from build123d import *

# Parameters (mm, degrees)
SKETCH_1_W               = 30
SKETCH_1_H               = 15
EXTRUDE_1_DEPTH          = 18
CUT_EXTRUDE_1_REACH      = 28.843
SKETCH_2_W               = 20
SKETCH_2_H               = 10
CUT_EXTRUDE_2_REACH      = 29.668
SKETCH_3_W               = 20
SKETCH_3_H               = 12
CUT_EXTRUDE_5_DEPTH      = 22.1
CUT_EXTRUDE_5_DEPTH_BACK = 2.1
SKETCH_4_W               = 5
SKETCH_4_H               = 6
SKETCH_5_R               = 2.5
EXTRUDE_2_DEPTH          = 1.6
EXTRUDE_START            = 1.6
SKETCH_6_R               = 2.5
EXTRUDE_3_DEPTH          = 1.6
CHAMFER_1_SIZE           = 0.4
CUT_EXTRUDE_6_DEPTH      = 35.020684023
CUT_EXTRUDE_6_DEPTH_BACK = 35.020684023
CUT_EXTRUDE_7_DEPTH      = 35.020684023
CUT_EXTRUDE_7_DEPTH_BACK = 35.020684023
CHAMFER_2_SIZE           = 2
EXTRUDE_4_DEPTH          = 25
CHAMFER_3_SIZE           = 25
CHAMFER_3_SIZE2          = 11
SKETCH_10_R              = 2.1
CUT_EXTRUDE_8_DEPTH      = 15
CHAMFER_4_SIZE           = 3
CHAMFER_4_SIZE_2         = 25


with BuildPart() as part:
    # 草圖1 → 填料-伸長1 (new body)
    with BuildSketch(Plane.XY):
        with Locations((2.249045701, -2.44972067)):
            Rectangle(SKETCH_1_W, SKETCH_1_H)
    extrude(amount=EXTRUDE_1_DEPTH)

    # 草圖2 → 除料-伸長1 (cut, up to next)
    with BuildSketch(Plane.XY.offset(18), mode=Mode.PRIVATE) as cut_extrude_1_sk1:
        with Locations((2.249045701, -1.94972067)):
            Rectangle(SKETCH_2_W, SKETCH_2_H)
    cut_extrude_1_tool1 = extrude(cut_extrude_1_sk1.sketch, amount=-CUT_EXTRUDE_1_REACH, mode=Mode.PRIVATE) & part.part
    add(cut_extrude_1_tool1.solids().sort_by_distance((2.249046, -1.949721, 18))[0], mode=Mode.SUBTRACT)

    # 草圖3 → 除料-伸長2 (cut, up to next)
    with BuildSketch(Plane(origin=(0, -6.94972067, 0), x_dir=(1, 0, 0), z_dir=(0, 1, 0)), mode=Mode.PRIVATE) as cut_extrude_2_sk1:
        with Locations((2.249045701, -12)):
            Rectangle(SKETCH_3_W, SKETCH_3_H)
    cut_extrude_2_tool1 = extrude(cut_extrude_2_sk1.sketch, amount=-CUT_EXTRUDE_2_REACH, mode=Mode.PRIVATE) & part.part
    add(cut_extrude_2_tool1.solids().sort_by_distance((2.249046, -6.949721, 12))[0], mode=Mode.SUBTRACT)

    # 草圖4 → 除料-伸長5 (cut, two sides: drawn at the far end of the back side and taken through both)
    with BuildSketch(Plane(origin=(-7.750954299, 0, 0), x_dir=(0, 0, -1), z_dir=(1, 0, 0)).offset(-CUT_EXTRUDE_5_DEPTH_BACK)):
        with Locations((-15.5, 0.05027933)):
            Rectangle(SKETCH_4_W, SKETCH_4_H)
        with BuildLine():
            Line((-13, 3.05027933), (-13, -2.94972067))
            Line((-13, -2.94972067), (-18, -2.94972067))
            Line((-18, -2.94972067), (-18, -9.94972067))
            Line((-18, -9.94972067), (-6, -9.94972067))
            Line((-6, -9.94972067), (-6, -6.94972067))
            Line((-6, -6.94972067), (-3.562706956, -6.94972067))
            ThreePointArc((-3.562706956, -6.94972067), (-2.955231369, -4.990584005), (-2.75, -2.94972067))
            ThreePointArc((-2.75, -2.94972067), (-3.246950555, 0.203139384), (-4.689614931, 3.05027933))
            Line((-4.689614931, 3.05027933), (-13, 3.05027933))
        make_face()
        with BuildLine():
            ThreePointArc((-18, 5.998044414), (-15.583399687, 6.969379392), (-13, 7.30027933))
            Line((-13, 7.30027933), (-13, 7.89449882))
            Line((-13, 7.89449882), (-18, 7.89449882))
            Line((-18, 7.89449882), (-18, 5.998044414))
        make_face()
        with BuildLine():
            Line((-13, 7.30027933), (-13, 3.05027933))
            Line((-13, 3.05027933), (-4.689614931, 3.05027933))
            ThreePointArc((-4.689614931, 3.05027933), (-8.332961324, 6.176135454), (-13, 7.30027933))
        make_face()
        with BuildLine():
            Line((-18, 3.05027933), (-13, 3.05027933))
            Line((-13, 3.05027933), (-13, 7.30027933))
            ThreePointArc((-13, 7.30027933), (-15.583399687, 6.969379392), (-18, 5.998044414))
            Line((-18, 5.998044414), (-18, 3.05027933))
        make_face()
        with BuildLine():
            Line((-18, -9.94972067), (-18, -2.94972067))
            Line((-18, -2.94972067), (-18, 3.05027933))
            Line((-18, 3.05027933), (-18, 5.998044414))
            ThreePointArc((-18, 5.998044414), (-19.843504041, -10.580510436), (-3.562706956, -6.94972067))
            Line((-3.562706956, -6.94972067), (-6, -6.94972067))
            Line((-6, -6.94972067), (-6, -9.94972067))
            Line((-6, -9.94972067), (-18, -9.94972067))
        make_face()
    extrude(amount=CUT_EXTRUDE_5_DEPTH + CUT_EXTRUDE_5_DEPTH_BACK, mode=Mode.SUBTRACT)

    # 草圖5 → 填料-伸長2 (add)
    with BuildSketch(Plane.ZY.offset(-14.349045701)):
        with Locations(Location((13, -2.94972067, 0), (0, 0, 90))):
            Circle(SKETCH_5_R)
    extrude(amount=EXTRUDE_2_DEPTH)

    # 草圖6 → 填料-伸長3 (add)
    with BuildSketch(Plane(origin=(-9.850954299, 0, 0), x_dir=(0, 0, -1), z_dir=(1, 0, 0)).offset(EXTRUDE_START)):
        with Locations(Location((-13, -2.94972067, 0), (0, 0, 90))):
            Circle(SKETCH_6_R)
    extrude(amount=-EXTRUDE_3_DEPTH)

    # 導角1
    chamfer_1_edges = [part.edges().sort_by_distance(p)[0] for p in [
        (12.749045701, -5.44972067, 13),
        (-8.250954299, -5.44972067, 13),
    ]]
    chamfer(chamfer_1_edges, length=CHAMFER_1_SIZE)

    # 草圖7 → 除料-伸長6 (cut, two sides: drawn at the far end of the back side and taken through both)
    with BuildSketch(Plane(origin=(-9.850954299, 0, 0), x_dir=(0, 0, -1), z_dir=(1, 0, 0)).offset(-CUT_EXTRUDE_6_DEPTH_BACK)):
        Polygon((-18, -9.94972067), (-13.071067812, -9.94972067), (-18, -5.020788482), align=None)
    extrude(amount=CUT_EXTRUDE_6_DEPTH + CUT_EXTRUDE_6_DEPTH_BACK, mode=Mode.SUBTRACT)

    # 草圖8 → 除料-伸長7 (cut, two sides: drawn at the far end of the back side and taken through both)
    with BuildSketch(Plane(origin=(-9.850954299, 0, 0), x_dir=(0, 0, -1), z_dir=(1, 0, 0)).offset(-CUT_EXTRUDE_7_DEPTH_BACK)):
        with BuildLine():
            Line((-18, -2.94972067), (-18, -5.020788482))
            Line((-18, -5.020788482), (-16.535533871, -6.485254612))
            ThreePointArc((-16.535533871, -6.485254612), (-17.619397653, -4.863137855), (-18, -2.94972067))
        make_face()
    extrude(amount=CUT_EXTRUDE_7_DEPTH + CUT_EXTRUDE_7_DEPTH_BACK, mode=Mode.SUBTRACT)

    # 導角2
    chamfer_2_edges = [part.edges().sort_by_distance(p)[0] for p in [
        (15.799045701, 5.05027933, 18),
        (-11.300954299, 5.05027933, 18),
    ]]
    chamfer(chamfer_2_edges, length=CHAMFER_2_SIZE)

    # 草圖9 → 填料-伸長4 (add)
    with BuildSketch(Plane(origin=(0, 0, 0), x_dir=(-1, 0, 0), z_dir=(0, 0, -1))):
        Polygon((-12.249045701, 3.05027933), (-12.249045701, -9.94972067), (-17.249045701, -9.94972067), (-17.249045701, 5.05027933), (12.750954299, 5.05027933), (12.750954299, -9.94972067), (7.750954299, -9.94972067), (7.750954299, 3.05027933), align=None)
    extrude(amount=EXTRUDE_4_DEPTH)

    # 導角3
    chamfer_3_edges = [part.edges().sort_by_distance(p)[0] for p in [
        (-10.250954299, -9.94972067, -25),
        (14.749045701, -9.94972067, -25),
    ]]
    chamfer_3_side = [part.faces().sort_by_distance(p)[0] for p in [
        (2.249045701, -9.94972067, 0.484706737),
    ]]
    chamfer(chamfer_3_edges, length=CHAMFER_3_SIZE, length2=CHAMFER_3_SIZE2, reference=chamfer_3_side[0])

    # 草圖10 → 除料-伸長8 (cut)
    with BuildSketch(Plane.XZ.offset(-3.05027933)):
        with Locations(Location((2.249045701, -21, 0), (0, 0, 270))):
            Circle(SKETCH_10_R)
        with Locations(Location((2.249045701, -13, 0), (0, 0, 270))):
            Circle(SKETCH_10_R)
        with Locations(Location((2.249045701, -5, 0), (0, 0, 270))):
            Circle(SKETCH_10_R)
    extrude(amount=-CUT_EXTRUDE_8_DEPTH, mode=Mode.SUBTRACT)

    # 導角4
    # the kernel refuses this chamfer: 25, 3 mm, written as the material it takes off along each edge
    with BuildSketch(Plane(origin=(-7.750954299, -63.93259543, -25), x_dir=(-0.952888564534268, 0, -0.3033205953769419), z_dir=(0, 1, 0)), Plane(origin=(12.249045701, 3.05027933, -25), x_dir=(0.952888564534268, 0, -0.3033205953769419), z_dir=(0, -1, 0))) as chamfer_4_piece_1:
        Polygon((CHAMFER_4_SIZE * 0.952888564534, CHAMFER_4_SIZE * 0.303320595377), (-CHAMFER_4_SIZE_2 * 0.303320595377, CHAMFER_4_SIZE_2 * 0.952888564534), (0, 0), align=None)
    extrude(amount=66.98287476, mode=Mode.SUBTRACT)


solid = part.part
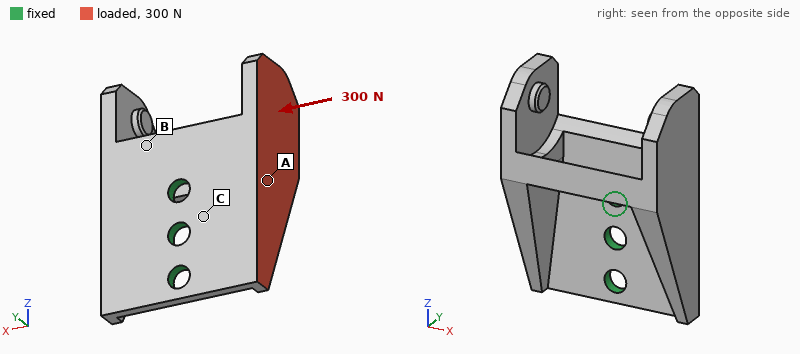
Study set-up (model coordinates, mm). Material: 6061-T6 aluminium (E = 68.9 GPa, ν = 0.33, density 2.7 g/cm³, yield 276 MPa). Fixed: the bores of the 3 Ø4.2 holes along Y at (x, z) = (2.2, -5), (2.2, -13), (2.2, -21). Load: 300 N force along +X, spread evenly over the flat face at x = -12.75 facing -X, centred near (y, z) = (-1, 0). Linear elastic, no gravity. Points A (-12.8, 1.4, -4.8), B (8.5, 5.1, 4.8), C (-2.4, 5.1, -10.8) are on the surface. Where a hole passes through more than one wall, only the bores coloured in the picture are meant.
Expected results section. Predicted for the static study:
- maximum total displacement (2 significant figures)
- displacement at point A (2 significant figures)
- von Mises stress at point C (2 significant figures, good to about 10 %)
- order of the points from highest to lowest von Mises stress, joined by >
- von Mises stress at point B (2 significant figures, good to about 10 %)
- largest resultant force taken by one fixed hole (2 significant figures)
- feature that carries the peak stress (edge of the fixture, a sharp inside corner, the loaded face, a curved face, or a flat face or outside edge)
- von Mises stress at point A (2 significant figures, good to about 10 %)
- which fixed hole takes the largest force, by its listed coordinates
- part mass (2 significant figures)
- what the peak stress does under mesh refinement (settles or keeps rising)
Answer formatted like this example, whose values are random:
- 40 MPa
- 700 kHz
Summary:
- 0.10 mm
- 0.046 mm
- 32 MPa
- C > B > A
- 24 MPa
- 320 N
- edge of the fixture
- 7.2 MPa
- (2.2, -5)
- 14 g
- keeps rising
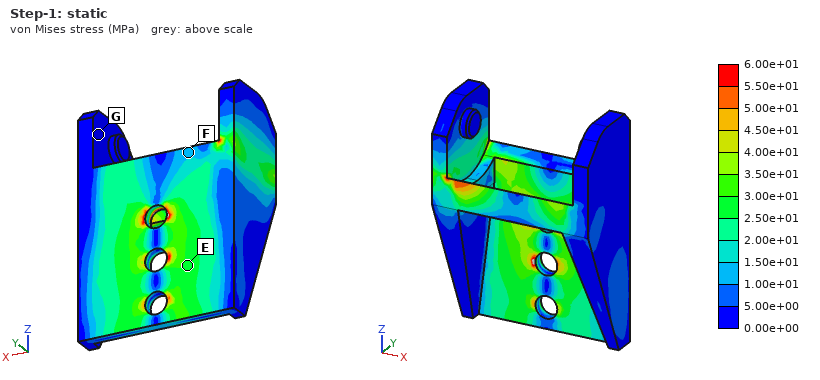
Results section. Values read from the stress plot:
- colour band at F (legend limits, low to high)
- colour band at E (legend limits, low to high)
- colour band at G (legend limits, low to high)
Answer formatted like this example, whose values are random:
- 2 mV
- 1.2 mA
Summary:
- 1.00e+01 to 1.50e+01 MPa
- 2.50e+01 to 3.00e+01 MPa
- 0.00e+00 to 5.00e+00 MPa
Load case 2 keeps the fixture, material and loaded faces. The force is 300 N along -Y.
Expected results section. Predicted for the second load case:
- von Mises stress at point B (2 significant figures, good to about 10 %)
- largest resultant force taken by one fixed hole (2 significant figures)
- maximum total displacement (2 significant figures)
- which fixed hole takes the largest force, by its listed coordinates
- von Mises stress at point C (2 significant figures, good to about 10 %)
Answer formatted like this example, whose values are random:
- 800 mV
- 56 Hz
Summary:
- 29 MPa
- 320 N
- 0.24 mm
- (2.2, -5)
- 98 MPa
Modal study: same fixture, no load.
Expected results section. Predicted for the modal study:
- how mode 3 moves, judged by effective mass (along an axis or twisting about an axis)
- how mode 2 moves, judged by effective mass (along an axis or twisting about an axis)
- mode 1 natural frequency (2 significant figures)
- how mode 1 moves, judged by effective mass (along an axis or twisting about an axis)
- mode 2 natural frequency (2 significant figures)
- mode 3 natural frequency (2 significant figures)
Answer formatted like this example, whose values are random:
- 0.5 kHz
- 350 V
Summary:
- along X
- along Y
- 2400 Hz
- along X
- 3600 Hz
- 5600 Hz
